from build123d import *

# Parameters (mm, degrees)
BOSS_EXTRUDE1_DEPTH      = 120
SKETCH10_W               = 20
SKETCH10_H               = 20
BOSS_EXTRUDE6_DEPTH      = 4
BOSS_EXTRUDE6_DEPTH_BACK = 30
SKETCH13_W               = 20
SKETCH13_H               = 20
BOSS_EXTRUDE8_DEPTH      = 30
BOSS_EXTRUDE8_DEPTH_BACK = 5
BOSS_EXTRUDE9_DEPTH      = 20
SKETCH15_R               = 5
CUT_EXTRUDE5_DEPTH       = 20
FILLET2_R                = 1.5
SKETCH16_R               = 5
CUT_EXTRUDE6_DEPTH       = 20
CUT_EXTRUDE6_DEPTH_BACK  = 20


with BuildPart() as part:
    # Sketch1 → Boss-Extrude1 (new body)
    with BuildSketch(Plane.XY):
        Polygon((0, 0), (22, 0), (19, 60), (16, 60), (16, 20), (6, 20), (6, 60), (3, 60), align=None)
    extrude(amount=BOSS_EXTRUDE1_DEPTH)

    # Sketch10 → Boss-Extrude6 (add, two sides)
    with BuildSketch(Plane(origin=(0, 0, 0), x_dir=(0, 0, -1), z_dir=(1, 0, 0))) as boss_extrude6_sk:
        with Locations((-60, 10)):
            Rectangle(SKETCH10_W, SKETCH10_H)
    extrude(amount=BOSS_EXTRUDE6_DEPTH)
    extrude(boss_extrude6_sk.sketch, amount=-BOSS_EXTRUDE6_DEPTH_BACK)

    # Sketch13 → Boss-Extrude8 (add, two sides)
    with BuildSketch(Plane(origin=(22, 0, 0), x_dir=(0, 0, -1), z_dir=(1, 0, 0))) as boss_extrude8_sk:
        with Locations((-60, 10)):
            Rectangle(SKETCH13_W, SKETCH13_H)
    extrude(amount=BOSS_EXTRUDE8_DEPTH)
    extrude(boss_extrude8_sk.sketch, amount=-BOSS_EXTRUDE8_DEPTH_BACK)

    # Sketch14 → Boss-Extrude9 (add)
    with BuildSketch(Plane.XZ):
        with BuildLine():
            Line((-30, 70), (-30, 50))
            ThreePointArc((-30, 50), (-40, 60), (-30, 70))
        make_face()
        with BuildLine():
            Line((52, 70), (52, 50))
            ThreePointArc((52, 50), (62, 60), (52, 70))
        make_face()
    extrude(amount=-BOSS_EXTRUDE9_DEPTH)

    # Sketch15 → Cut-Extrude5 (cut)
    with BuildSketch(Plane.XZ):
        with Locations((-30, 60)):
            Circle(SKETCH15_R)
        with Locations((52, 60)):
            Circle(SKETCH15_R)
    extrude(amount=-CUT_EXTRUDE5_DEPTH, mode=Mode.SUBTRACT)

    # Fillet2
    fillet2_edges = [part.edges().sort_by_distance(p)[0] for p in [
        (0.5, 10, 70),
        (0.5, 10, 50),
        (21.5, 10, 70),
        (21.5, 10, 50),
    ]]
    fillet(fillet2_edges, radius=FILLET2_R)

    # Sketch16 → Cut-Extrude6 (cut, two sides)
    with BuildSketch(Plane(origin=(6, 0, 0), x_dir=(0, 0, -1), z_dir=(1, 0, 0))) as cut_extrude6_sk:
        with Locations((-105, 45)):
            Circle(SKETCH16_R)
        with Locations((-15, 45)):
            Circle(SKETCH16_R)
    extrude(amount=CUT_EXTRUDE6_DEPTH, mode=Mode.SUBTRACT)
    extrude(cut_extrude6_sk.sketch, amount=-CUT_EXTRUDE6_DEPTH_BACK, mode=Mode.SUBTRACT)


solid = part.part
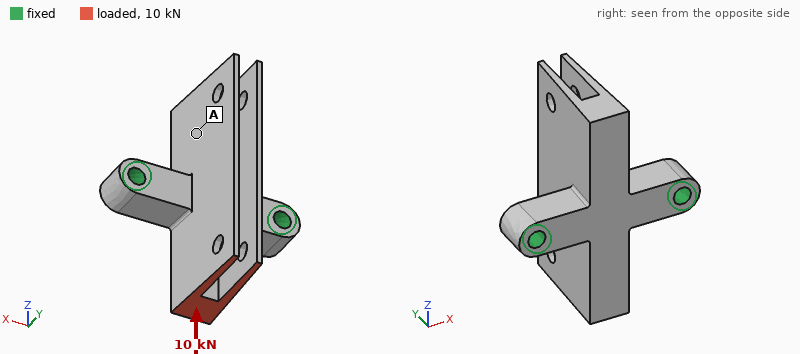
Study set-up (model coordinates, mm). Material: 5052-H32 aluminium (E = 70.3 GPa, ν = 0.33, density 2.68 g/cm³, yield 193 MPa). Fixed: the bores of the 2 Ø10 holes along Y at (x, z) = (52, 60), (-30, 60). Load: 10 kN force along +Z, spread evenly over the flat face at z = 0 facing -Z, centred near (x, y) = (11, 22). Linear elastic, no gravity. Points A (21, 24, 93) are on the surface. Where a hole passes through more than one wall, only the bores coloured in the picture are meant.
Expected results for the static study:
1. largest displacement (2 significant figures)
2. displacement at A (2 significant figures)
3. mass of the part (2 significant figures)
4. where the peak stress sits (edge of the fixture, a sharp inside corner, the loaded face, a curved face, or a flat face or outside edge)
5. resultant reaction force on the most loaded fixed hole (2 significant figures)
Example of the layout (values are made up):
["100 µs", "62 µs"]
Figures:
["0.30 mm", "0.14 mm", "310 g", "a curved face", "5.0 kN"]
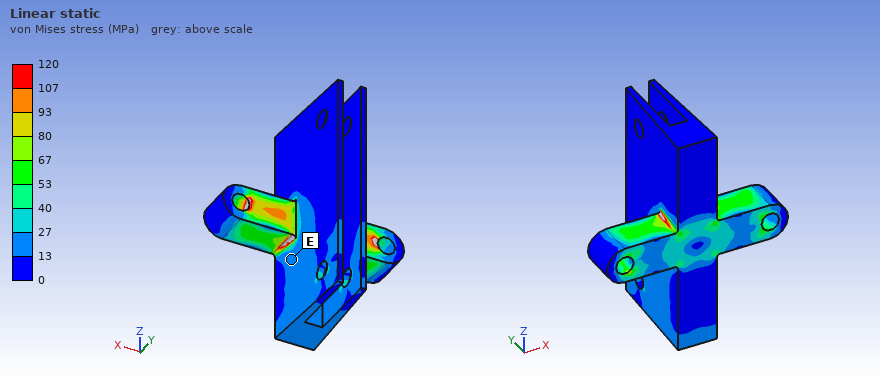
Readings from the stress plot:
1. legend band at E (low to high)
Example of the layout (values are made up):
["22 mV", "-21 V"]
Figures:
["13 to 27 MPa"]
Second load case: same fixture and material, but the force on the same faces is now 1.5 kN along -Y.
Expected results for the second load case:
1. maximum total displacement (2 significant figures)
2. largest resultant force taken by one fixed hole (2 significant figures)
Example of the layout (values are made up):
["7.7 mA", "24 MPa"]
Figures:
["0.21 mm", "770 N"]
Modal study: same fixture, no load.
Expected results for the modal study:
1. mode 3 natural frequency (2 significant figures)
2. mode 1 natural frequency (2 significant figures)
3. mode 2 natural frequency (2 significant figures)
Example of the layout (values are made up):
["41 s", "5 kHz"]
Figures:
["2400 Hz", "1600 Hz", "2300 Hz"]
